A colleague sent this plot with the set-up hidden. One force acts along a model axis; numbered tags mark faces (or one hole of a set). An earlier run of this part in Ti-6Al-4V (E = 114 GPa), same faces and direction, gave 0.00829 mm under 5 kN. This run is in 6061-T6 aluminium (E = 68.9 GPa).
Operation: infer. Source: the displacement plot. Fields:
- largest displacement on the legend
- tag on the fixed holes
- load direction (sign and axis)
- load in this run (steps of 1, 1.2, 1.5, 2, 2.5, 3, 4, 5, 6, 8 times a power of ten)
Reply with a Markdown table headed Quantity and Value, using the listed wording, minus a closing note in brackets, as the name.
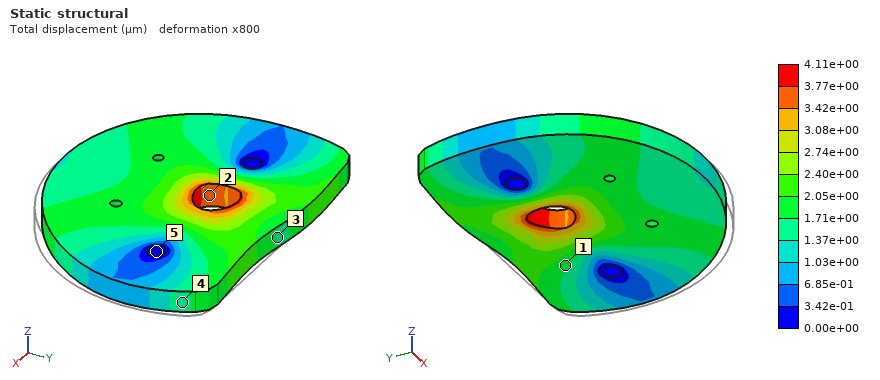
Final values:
| Quantity | Value |
|---|---|
| largest displacement on the legend | 4.11e+00 µm |
| tag on the fixed holes | 5 |
| load direction | -X |
| load in this run | 1.5 kN |
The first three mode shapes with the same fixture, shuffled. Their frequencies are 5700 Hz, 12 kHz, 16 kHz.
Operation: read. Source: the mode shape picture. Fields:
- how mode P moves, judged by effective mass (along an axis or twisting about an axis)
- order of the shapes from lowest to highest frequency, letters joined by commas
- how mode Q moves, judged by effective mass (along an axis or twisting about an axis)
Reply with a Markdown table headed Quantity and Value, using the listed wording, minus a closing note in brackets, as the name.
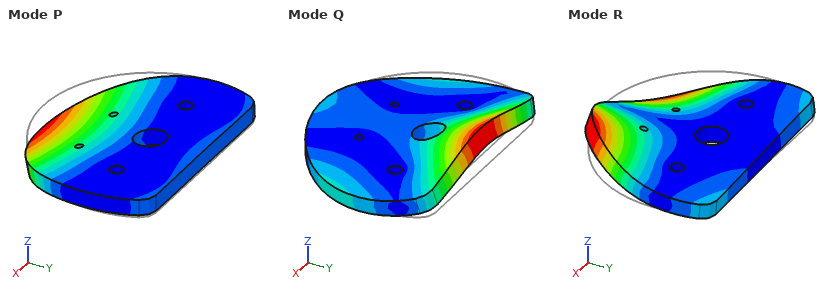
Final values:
| Quantity | Value |
|---|---|
| how mode P moves, judged by effective mass | along Z |
| order of the shapes from lowest to highest frequency, letters joined by commas | P, R, Q |
| how mode Q moves, judged by effective mass | along Z |
